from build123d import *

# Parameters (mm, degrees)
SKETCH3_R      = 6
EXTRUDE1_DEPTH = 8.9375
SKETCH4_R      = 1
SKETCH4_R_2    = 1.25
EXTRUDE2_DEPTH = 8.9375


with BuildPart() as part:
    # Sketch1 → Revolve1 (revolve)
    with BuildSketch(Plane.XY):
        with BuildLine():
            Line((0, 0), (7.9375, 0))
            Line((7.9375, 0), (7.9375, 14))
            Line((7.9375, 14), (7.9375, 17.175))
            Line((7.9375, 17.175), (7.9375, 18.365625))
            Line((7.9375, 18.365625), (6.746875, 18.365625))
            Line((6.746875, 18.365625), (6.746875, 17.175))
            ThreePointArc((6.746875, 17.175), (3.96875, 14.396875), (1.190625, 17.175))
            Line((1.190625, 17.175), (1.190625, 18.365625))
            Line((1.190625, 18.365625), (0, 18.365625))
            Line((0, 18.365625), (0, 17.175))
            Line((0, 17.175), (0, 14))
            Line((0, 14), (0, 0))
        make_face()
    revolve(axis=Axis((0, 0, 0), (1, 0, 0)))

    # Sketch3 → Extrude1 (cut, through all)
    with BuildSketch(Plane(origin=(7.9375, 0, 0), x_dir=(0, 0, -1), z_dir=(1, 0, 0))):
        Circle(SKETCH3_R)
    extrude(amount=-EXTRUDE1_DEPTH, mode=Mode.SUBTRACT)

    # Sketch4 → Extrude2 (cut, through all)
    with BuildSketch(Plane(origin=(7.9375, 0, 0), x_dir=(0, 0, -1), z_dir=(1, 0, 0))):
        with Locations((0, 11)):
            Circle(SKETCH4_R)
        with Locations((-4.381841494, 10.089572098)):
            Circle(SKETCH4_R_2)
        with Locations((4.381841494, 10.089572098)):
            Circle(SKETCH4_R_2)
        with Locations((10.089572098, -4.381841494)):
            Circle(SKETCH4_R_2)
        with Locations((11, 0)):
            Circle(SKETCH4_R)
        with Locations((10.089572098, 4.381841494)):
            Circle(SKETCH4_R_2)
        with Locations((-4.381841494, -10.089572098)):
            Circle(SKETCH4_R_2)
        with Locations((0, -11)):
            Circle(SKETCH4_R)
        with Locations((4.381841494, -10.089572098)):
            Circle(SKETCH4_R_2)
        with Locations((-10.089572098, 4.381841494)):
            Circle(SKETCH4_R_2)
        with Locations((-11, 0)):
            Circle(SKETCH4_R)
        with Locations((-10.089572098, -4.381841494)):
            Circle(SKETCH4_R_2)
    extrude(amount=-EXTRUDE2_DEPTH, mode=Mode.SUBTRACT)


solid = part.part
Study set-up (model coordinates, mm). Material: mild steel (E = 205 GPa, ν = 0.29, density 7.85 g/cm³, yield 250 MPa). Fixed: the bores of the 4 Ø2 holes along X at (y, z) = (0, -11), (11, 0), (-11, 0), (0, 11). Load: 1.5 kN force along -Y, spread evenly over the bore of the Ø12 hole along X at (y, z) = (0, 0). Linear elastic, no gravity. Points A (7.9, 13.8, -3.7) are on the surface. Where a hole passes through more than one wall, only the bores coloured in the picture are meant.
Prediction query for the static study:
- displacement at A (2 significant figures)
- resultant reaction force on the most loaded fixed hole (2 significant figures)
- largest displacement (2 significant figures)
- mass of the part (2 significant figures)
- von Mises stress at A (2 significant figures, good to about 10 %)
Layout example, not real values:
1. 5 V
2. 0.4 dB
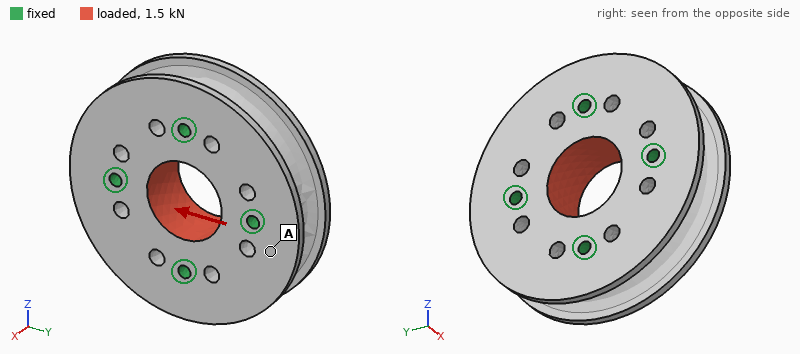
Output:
1. 0.078 µm
2. 420 N
3. 0.33 µm
4. 40 g
5. 1.8 MPa
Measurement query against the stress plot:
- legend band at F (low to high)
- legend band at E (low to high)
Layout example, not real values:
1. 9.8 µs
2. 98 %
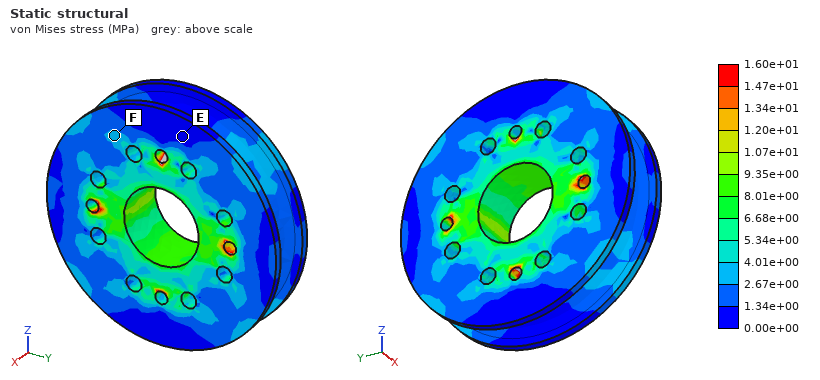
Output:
1. 2.67e+00 to 4.01e+00 MPa
2. 0.00e+00 to 1.34e+00 MPa
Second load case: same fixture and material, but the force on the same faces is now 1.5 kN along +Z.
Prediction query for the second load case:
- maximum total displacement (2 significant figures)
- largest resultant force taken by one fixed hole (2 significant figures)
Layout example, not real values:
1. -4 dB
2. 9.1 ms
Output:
1. 0.33 µm
2. 420 N
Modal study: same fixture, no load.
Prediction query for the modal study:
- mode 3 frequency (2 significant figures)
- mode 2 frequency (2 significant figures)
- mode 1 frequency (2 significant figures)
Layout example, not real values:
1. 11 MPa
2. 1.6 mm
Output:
1. 43 kHz
2. 43 kHz
3. 40 kHz
